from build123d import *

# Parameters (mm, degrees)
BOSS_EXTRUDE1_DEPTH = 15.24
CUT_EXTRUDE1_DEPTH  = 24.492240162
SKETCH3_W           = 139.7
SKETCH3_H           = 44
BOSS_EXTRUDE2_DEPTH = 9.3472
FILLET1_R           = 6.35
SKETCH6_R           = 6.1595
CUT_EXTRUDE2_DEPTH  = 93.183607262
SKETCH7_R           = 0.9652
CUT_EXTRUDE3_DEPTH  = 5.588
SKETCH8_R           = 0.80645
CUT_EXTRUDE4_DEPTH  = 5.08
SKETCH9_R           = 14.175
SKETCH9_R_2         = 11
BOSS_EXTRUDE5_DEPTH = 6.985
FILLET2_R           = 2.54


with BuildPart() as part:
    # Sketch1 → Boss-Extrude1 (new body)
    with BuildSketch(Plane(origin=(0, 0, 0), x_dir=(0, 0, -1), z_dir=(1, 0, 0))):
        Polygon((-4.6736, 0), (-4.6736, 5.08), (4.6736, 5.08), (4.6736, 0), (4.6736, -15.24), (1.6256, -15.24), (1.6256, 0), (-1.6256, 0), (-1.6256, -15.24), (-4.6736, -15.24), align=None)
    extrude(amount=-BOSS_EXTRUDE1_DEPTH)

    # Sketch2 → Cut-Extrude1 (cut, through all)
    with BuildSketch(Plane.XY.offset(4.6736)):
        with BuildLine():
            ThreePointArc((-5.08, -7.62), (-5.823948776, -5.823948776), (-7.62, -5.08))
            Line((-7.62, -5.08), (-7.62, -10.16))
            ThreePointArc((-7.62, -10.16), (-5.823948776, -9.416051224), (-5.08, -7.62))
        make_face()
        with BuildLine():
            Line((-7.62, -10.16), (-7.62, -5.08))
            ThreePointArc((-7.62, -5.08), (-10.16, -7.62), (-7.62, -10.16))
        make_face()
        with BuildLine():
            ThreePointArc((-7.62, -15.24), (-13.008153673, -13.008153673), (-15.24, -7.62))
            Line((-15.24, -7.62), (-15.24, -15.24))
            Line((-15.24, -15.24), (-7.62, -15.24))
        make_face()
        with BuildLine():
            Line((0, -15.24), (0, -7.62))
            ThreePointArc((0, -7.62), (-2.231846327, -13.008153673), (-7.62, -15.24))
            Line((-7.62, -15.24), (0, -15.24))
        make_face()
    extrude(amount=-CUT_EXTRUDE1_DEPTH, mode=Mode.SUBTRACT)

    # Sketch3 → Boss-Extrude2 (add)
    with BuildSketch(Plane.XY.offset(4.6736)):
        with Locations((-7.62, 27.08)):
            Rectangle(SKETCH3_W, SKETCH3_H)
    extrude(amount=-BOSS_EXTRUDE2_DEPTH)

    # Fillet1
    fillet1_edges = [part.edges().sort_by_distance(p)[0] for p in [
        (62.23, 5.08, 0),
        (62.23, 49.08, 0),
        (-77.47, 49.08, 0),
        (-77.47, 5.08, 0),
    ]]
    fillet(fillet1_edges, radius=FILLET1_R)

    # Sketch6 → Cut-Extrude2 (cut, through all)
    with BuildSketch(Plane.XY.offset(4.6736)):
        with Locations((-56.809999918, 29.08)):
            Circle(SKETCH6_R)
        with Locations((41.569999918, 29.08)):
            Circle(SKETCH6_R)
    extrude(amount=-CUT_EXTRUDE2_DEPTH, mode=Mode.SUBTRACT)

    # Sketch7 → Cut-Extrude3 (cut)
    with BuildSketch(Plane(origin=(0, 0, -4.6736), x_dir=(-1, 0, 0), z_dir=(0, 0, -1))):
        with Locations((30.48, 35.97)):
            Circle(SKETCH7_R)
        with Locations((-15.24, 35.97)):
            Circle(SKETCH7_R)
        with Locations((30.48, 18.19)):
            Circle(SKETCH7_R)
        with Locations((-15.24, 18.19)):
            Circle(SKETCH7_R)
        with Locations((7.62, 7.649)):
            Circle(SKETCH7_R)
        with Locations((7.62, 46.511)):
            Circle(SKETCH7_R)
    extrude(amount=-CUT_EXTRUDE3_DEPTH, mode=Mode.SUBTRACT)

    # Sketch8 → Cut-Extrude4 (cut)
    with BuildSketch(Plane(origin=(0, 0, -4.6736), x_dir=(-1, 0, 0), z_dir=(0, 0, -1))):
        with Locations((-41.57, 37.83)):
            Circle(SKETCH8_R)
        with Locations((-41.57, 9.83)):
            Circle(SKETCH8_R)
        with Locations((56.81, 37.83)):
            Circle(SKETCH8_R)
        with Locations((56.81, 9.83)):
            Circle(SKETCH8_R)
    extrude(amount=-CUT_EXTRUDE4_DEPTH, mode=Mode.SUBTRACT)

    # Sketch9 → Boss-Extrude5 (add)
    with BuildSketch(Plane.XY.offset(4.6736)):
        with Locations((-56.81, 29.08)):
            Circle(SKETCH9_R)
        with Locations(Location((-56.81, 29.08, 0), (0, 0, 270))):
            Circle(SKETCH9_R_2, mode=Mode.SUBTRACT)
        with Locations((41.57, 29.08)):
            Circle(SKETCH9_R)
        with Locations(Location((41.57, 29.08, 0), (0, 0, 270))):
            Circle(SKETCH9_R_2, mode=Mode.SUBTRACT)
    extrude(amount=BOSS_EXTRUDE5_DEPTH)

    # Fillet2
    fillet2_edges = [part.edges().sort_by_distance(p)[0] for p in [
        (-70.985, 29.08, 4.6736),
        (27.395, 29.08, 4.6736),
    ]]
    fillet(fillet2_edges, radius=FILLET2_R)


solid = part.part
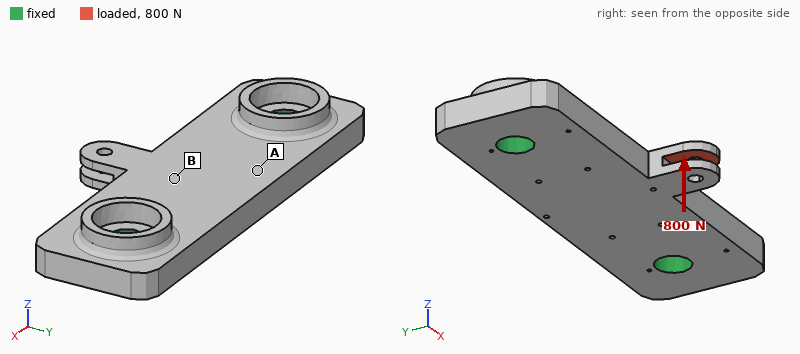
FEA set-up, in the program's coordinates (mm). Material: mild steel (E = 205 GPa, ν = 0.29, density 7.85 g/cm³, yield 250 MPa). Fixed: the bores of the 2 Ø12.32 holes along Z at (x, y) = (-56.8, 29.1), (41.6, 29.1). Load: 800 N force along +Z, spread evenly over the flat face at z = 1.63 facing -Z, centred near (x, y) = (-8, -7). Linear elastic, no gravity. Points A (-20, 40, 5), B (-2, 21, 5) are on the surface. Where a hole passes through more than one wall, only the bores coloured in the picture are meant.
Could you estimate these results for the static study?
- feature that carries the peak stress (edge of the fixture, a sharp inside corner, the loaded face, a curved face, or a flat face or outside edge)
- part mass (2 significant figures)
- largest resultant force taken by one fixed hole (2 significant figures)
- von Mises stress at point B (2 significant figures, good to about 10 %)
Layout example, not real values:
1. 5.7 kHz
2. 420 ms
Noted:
1. a flat face or outside edge
2. 470 g
3. 400 N
4. 25 MPa
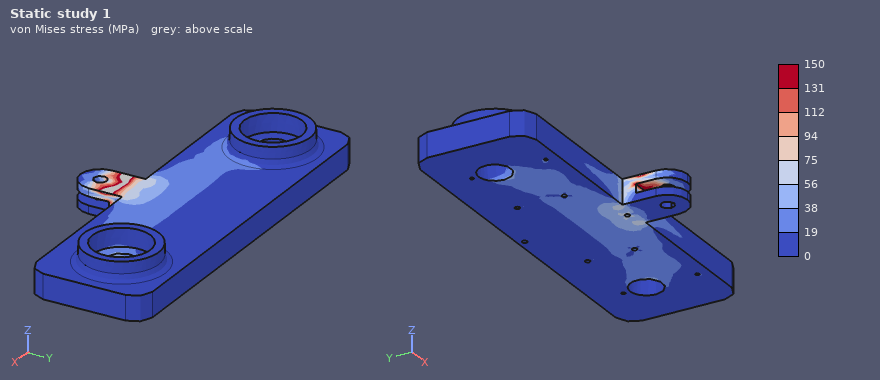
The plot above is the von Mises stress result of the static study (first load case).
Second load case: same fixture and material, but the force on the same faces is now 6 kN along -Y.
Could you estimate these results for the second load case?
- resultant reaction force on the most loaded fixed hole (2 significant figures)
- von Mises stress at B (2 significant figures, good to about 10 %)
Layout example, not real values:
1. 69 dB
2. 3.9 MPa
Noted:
1. 3.1 kN
2. 26 MPa
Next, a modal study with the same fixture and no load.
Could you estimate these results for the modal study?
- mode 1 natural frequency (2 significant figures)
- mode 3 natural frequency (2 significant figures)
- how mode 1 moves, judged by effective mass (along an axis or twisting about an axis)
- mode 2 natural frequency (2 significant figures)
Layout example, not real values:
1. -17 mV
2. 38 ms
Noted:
1. 4500 Hz
2. 10 kHz
3. along Z
4. 6200 Hz
